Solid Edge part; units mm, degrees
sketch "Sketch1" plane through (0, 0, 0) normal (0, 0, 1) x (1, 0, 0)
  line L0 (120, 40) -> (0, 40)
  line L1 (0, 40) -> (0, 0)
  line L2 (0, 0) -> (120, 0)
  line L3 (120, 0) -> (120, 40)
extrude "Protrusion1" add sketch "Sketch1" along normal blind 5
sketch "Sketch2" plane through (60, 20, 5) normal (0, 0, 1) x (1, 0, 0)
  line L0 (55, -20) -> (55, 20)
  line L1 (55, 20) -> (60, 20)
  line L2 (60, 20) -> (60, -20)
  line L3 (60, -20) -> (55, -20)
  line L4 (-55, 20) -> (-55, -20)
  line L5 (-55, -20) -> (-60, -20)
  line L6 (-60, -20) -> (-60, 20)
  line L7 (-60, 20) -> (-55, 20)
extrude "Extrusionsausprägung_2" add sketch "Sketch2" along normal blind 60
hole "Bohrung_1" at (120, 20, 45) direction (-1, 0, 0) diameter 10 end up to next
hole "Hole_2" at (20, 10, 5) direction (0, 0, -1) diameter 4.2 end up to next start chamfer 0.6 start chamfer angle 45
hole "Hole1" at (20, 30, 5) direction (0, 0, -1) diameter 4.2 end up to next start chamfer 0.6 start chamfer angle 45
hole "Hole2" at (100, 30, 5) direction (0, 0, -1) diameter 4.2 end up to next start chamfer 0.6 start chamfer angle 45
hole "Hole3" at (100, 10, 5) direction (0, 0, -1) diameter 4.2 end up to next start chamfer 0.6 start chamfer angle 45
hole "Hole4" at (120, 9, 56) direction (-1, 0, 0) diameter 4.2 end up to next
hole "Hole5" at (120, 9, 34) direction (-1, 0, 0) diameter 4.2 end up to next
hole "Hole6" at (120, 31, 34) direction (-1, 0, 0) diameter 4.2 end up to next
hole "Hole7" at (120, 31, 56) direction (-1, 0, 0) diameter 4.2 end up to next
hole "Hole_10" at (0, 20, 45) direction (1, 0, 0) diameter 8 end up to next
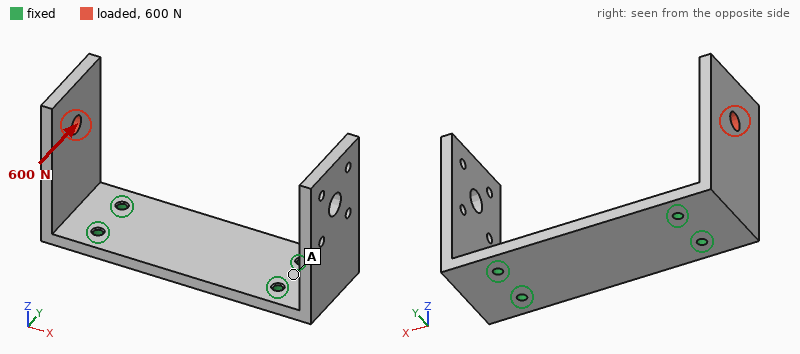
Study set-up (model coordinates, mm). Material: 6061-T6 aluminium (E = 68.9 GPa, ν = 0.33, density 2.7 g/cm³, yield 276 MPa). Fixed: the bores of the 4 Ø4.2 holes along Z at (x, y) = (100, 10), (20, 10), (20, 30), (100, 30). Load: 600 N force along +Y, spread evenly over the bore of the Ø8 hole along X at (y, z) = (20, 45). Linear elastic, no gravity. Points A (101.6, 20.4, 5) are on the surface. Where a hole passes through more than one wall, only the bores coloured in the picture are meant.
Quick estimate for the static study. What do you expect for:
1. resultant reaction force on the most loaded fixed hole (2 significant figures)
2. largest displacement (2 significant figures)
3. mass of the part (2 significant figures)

1.1 kN
0.32 mm
130 g
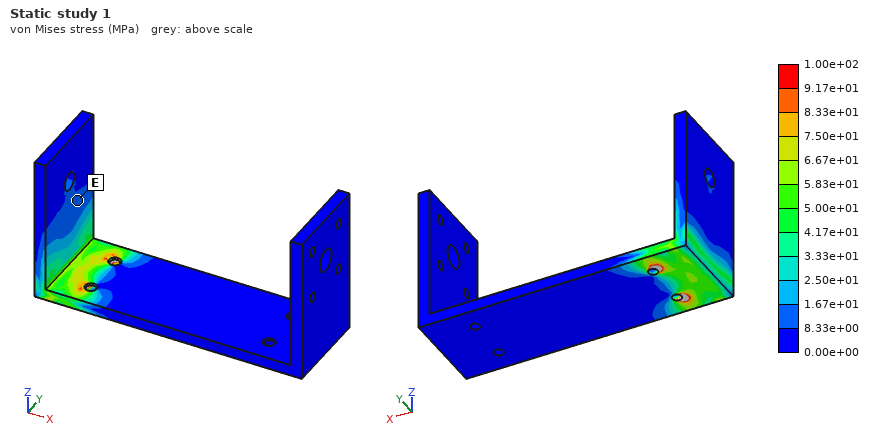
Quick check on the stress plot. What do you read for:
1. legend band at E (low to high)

8.33e+00 to 1.67e+01 MPa
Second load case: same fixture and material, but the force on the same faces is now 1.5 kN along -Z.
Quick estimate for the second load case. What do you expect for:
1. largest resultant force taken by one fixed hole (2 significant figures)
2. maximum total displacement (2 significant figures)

770 N
0.53 mm
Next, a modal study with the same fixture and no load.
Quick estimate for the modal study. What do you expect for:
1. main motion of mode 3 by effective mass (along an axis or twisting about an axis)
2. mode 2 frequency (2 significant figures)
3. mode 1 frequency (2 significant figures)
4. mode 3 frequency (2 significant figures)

along Y
770 Hz
750 Hz
1700 Hz
